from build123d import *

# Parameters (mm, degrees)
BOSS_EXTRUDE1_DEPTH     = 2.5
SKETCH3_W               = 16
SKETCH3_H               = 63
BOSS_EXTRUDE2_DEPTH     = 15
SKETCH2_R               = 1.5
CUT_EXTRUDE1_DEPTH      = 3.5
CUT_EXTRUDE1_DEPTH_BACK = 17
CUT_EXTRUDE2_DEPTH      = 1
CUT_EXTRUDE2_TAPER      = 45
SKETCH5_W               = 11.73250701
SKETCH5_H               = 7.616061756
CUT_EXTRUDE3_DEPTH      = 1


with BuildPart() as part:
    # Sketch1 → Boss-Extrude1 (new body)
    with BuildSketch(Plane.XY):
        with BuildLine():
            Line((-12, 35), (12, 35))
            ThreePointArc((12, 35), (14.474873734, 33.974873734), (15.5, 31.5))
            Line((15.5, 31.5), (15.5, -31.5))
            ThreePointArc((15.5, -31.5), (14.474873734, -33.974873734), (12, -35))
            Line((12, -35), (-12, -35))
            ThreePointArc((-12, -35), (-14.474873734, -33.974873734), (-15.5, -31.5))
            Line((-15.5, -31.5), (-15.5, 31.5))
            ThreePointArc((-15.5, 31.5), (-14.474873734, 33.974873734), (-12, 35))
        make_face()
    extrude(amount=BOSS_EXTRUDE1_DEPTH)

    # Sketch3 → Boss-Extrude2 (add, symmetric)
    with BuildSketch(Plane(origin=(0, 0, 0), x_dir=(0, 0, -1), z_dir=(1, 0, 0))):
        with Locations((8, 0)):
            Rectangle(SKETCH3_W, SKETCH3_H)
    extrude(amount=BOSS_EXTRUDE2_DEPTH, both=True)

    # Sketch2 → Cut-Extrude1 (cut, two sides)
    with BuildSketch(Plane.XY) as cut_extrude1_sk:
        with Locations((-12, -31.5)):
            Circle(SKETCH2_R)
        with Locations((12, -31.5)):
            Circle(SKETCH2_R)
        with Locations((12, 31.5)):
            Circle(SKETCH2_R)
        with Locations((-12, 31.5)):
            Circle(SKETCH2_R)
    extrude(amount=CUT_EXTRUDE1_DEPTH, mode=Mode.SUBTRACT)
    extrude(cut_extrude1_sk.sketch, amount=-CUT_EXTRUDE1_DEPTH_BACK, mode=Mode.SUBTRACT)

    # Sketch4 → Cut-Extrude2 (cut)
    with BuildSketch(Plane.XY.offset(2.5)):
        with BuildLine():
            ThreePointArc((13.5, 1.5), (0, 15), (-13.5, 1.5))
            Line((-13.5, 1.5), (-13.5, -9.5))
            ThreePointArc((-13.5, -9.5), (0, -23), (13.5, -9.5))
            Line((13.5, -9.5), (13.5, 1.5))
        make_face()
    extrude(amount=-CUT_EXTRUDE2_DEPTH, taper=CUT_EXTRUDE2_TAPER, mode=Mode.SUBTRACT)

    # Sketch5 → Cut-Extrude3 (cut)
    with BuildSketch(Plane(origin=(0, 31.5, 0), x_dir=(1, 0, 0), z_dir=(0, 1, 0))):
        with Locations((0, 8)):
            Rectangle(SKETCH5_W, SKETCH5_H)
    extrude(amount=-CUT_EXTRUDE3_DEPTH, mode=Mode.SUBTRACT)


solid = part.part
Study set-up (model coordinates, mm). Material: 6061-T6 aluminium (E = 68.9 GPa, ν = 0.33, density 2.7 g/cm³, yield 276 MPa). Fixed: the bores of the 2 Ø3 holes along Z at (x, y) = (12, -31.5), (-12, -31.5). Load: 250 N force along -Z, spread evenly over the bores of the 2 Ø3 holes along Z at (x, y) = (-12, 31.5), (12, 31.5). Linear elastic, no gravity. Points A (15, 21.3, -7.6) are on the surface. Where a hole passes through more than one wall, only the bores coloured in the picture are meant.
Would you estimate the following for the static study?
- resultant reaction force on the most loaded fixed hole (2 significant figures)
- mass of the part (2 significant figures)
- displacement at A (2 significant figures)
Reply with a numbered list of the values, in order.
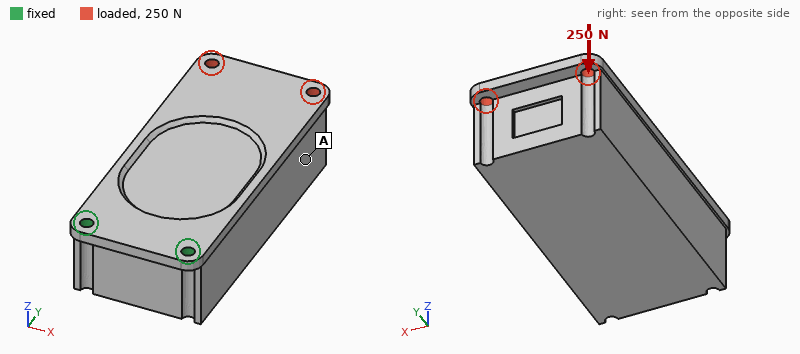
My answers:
1. 130 N
2. 93 g
3. 0.66 mm
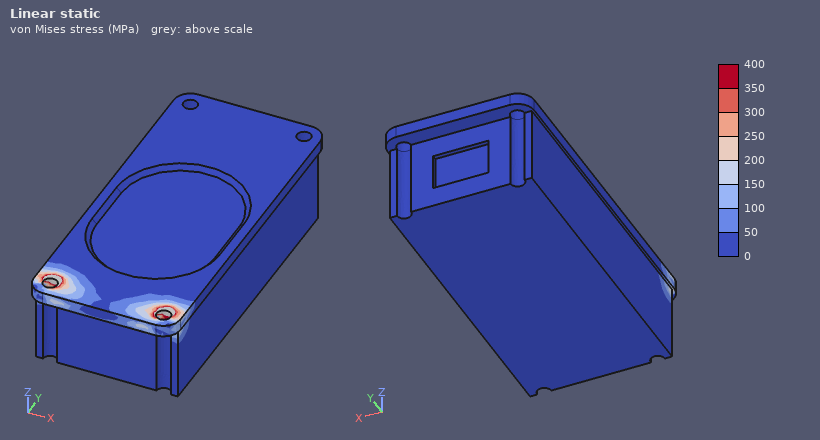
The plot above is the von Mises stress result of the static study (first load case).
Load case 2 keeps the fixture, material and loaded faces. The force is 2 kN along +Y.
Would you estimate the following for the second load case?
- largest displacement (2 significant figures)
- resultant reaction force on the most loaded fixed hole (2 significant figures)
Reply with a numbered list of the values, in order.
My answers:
1. 77 µm
2. 1.0 kN
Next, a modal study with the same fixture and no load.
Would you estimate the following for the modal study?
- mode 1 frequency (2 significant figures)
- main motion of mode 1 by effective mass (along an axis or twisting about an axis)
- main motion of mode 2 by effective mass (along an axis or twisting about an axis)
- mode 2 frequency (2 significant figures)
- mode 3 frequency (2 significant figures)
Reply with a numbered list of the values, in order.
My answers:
1. 500 Hz
2. along Z
3. along X
4. 3200 Hz
5. 7600 Hz
